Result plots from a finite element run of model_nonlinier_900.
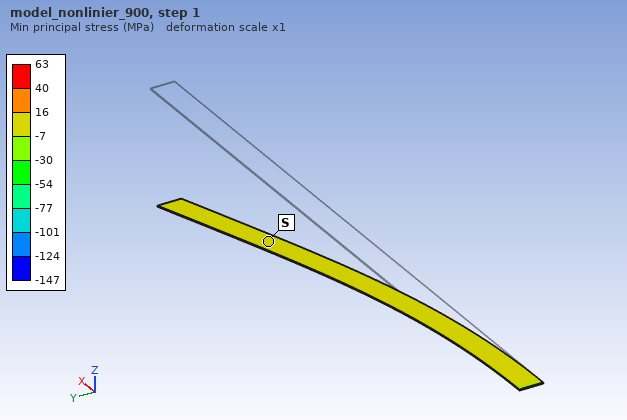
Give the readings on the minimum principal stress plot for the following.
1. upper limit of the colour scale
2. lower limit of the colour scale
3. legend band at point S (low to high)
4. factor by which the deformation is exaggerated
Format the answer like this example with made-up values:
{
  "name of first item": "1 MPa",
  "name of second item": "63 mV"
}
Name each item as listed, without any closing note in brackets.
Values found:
{
  "upper limit of the colour scale": "63 MPa",
  "lower limit of the colour scale": "-147 MPa",
  "legend band at point S": "-7 to 16 MPa",
  "factor by which the deformation is exaggerated": "1"
}
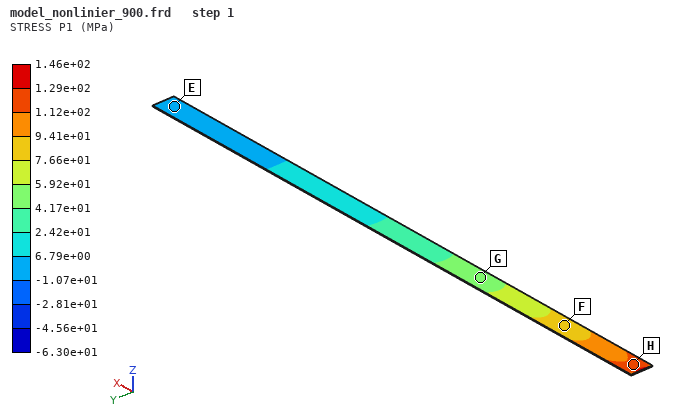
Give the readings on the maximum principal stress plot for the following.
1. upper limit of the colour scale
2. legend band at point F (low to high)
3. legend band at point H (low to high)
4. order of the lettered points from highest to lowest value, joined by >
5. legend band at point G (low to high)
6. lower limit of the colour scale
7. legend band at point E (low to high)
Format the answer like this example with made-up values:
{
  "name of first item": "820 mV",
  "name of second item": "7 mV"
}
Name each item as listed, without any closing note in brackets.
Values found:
{
  "upper limit of the colour scale": "1.46e+02 MPa",
  "legend band at point F": "7.66e+01 to 9.41e+01 MPa",
  "legend band at point H": "1.12e+02 to 1.29e+02 MPa",
  "order of the lettered points from highest to lowest value, joined by >": "H > F > G > E",
  "legend band at point G": "4.17e+01 to 5.92e+01 MPa",
  "lower limit of the colour scale": "-6.30e+01 MPa",
  "legend band at point E": "-1.07e+01 to 6.79e+00 MPa"
}
